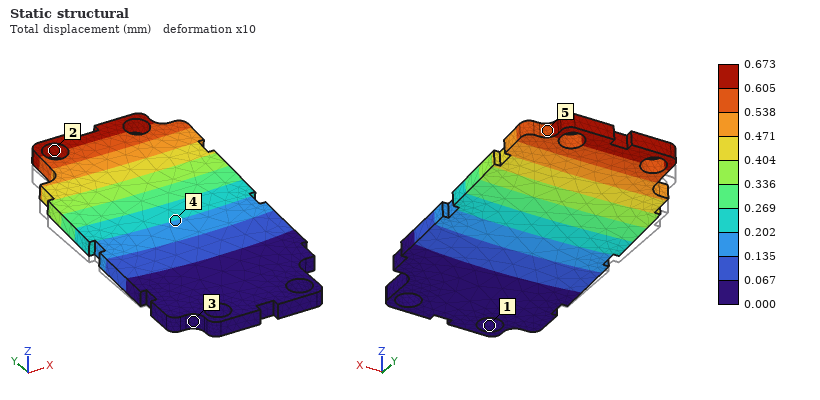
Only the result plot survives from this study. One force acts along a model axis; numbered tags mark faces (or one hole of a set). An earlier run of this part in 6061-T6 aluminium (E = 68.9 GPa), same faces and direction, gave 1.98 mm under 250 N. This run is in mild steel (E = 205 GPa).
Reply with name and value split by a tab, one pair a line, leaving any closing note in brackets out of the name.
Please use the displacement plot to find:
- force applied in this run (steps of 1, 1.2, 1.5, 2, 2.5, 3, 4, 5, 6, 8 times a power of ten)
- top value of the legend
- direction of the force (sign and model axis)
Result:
force applied in this run	250 N
top value of the legend	0.673 mm
direction of the force	+Z
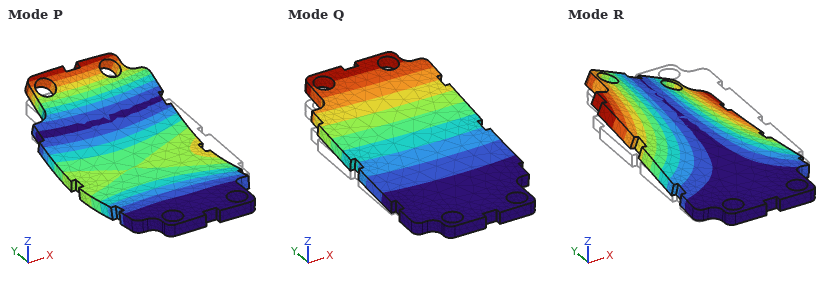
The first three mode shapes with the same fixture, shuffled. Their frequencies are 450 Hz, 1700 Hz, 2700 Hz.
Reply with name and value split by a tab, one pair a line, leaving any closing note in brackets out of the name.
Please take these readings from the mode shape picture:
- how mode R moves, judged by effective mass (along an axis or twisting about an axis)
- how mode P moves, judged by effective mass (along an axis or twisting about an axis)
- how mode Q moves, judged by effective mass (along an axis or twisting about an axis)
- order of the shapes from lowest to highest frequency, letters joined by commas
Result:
how mode R moves, judged by effective mass	twisting about Y
how mode P moves, judged by effective mass	along Z
how mode Q moves, judged by effective mass	along Z
order of the shapes from lowest to highest frequency, letters joined by commas	Q, R, P
